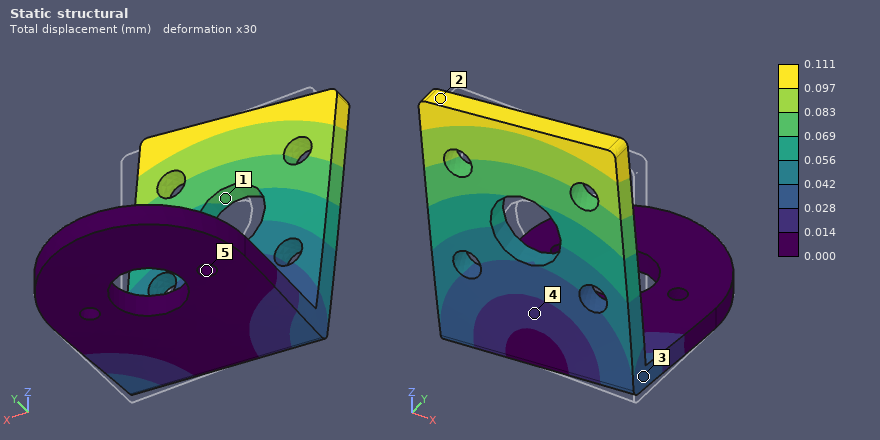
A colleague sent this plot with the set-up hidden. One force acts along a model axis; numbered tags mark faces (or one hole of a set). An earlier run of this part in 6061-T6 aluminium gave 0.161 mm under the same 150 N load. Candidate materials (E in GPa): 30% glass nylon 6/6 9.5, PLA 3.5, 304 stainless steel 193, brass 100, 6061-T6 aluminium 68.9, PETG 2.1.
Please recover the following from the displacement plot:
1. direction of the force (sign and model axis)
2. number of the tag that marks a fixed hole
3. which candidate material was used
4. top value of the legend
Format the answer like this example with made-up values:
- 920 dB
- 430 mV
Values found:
- -X
- 5
- brass
- 0.111 mm
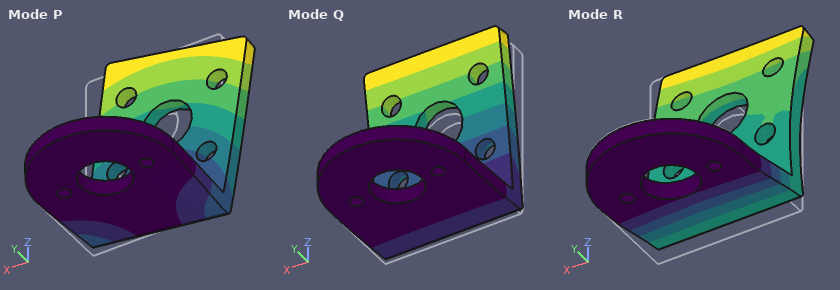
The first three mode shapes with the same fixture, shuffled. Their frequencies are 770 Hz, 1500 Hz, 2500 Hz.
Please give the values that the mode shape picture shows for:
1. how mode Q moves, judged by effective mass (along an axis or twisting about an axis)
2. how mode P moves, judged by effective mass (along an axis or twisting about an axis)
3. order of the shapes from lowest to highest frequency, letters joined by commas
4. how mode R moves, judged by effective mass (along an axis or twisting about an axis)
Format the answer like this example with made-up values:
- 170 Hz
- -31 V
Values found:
- along Y
- along X
- Q, P, R
- along Z
